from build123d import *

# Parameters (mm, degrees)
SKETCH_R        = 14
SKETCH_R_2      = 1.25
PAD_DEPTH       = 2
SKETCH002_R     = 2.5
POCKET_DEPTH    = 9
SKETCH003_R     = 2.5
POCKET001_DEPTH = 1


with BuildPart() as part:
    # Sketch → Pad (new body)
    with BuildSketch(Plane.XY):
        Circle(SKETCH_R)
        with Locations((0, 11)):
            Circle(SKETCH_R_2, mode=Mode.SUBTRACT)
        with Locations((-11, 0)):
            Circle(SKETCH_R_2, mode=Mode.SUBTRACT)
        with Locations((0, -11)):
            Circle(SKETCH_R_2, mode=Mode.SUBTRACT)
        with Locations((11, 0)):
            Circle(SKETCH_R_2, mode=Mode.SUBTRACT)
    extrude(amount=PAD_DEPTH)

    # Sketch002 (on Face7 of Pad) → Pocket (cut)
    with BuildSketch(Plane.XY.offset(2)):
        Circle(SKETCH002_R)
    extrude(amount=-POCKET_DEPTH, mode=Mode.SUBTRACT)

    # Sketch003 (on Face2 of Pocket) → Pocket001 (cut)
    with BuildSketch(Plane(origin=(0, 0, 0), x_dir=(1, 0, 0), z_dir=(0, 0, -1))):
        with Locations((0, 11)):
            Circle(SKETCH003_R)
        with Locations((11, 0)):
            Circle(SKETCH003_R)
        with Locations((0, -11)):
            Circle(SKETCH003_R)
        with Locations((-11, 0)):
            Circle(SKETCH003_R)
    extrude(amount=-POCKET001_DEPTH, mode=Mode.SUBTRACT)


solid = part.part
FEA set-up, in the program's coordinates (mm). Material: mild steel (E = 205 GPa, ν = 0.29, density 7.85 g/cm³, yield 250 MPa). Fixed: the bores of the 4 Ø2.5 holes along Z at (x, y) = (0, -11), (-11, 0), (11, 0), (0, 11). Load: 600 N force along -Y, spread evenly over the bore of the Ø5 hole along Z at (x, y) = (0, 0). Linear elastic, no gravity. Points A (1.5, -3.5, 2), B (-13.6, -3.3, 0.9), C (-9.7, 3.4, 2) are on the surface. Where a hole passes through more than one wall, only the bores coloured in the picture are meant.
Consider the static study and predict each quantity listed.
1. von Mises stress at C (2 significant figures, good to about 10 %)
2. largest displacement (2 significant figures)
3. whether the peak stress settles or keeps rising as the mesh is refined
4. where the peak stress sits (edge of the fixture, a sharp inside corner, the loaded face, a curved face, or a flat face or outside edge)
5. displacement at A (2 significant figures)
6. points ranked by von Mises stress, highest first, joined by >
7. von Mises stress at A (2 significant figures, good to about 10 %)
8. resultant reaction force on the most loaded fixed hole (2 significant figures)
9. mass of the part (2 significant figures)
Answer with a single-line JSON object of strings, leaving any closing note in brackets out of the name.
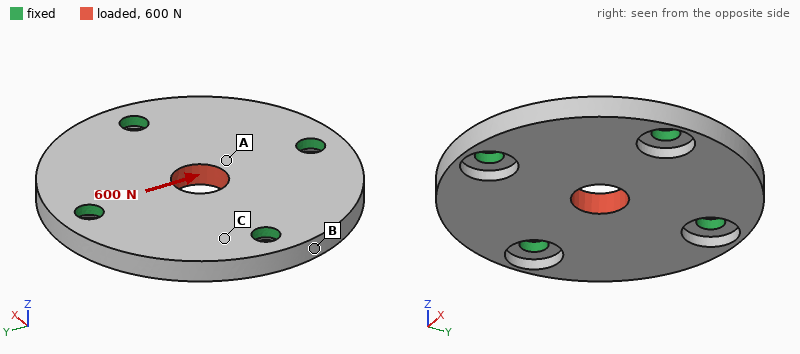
{"von Mises stress at C": "11 MPa", "largest displacement": "0.93 µm", "whether the peak stress settles or keeps rising as the mesh is refined": "keeps rising", "where the peak stress sits": "edge of the fixture", "displacement at A": "0.76 µm", "points ranked by von Mises stress, highest first, joined by >": "A > C > B", "von Mises stress at A": "19 MPa", "resultant reaction force on the most loaded fixed hole": "190 N", "mass of the part": "8.6 g"}
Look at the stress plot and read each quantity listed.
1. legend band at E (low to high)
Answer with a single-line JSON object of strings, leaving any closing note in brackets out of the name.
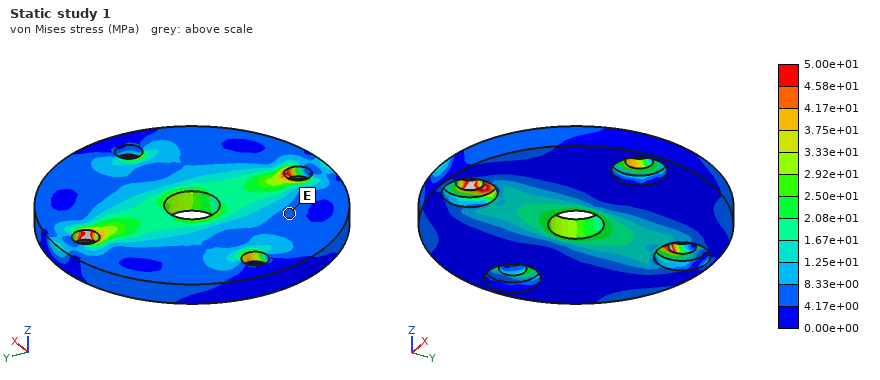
{"legend band at E": "4.17e+00 to 8.33e+00 MPa"}
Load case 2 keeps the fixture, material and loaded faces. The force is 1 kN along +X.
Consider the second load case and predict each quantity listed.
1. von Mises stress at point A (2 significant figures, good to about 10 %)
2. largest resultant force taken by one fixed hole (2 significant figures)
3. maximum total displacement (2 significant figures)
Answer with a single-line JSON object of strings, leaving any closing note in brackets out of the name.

{"von Mises stress at point A": "26 MPa", "largest resultant force taken by one fixed hole": "310 N", "maximum total displacement": "1.6 µm"}
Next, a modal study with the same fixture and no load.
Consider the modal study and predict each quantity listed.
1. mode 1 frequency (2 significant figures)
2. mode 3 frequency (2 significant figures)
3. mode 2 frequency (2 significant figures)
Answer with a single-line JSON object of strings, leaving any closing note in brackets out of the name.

{"mode 1 frequency": "24 kHz", "mode 3 frequency": "26 kHz", "mode 2 frequency": "26 kHz"}
